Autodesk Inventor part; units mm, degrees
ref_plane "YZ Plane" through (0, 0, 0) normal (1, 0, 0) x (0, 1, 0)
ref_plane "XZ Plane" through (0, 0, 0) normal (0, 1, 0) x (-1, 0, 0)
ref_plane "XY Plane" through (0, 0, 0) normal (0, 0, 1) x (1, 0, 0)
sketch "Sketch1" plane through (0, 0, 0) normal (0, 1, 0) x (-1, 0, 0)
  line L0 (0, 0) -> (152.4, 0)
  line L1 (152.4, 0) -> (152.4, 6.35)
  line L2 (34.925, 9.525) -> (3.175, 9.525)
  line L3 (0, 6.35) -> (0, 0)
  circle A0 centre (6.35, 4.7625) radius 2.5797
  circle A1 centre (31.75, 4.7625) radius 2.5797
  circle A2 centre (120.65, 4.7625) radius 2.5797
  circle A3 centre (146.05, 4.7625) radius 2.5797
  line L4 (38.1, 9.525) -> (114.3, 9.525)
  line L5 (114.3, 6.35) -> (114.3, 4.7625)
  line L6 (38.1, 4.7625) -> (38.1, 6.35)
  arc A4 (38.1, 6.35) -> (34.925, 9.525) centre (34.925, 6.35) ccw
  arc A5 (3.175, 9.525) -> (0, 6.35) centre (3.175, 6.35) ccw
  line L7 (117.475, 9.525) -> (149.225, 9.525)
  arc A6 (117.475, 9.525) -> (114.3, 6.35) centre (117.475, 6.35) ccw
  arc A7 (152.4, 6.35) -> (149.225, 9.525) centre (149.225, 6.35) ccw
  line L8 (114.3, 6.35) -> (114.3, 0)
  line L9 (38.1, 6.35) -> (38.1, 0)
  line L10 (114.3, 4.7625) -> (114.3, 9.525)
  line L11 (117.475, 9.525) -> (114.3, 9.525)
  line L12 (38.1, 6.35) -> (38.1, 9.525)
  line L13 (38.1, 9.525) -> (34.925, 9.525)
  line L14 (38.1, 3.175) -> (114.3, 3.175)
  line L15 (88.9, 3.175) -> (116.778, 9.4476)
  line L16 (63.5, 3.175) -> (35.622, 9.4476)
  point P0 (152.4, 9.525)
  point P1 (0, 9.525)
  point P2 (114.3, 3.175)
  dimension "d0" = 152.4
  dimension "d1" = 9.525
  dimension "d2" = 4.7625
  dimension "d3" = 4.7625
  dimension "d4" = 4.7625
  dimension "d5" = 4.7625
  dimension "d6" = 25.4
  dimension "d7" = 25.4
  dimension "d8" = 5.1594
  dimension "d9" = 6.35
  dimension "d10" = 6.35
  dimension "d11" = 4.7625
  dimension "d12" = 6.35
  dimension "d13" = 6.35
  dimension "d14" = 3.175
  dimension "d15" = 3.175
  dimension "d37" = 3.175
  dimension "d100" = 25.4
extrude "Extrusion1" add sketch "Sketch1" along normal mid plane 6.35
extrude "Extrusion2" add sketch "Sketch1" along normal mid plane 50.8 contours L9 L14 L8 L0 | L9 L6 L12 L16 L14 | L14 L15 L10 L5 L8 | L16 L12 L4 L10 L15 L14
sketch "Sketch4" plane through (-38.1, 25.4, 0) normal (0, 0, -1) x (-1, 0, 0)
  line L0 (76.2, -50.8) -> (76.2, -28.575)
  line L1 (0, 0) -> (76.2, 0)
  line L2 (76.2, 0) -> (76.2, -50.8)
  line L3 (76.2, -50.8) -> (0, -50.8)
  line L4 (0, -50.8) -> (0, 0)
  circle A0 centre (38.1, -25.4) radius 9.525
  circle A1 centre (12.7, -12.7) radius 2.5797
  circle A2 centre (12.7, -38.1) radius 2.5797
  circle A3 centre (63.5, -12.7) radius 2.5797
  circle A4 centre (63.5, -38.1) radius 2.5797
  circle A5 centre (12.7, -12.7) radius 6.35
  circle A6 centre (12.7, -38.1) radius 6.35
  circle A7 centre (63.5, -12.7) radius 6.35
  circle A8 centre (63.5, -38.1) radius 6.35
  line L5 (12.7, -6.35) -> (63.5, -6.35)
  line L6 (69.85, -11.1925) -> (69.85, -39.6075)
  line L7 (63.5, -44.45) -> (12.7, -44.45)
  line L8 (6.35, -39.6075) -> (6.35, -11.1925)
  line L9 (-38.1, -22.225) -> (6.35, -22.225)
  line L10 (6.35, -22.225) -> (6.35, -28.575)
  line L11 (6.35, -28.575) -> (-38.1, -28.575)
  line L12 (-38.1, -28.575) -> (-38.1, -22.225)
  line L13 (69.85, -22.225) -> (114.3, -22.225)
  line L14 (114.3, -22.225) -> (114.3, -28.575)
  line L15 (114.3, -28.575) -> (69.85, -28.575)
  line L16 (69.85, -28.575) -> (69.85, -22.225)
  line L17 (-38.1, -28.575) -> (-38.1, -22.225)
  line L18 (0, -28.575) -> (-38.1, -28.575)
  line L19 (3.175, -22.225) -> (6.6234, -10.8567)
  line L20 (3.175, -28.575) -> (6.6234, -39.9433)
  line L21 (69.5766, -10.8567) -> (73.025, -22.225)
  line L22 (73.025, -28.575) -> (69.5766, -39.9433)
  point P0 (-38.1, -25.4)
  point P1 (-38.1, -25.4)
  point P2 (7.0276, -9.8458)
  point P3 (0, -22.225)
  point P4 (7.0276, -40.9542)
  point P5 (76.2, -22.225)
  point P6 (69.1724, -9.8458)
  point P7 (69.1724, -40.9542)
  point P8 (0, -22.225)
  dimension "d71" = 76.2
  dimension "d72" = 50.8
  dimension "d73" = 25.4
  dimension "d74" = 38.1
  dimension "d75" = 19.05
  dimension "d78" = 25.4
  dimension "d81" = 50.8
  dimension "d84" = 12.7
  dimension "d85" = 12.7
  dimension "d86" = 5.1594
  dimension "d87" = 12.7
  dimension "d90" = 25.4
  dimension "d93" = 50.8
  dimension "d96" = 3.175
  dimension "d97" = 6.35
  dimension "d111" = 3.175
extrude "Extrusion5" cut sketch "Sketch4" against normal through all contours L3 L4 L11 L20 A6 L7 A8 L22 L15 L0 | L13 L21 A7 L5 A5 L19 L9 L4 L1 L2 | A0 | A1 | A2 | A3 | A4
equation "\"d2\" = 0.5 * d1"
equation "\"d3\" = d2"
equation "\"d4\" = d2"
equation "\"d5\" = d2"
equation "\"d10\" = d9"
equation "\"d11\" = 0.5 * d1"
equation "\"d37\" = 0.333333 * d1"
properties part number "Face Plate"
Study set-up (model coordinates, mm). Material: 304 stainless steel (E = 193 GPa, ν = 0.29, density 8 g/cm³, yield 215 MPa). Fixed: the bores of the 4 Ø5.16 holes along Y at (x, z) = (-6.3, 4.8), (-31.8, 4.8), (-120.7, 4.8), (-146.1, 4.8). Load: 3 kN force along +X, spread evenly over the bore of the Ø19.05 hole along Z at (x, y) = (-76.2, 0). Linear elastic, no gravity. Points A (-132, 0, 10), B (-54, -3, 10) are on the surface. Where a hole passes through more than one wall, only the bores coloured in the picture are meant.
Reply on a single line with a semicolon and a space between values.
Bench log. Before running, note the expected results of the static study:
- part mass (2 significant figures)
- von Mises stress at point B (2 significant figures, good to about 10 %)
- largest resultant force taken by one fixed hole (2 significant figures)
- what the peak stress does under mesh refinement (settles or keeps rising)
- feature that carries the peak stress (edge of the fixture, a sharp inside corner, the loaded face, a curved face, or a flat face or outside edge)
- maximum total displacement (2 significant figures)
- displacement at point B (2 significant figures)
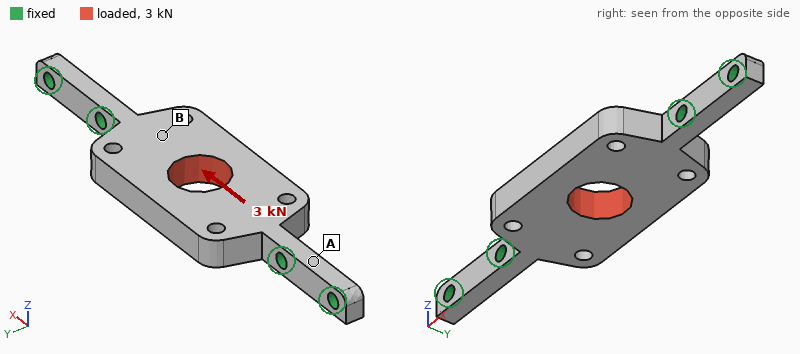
200 g; 8.7 MPa; 1.5 kN; keeps rising; edge of the fixture; 2.6 µm; 1.9 µm
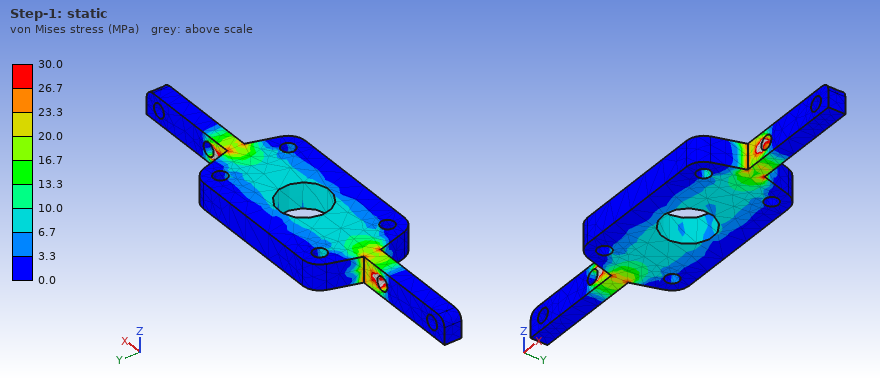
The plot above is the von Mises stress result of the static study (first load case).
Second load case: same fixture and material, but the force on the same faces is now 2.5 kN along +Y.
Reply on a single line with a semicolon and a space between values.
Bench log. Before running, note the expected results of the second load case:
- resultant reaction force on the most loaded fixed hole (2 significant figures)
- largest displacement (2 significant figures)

1.3 kN; 10 µm
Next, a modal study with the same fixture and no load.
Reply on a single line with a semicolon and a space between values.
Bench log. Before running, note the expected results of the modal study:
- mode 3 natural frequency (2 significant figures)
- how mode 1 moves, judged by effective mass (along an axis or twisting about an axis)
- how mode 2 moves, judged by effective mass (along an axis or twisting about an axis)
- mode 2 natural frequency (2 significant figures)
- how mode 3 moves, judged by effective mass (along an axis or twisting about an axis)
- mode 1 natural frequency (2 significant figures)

7100 Hz; twisting about X; along Z; 3600 Hz; along Y; 3000 Hz
